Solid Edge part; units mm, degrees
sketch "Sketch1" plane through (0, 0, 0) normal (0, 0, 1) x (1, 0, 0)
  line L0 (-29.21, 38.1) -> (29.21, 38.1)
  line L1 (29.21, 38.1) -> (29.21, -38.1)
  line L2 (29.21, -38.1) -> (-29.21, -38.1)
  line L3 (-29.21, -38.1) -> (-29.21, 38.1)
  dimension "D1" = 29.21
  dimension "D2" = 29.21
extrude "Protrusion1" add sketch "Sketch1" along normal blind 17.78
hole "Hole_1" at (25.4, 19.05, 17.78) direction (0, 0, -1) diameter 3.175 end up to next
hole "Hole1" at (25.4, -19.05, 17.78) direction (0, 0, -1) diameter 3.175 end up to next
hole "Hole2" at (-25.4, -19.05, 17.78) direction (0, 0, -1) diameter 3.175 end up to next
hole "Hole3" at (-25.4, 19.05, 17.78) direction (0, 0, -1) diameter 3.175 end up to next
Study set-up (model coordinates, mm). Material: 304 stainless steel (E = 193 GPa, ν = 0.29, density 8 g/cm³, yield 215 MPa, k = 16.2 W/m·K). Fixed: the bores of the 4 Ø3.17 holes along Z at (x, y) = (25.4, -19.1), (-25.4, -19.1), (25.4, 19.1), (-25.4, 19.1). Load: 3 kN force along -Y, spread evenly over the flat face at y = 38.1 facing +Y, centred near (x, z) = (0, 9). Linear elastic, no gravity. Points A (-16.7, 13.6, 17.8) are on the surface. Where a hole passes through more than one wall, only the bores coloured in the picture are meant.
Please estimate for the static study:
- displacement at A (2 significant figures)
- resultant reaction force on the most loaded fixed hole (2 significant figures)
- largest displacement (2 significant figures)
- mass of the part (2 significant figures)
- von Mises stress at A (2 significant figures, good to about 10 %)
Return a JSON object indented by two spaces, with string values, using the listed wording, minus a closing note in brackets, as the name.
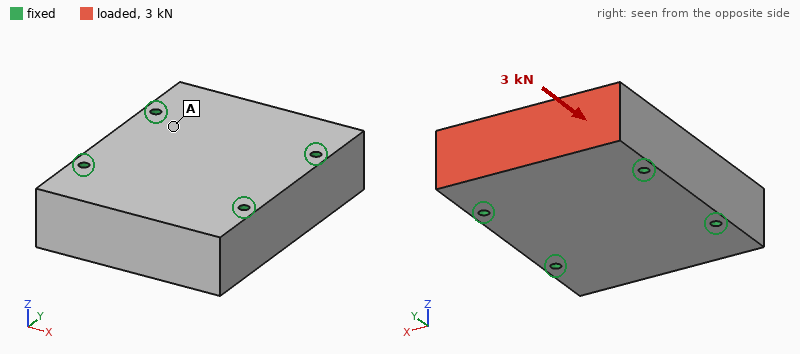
{
  "displacement at A": "0.23 µm",
  "resultant reaction force on the most loaded fixed hole": "1.1 kN",
  "largest displacement": "0.62 µm",
  "mass of the part": "630 g",
  "von Mises stress at A": "2.1 MPa"
}
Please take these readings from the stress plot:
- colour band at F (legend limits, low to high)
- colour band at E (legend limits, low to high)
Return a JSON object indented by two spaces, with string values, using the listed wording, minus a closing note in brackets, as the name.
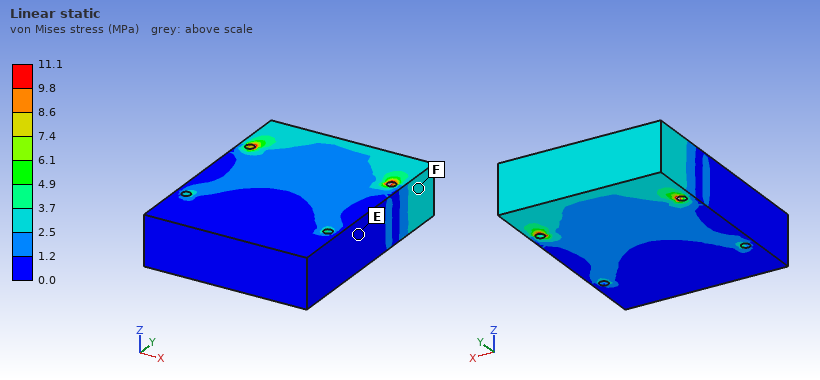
{
  "colour band at F": "2.5 to 3.7 MPa",
  "colour band at E": "0.0 to 1.2 MPa"
}
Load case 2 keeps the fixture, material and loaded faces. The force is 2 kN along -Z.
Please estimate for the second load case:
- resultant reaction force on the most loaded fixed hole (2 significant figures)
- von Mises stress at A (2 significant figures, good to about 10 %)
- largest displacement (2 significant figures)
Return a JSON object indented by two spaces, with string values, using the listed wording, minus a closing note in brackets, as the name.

{
  "resultant reaction force on the most loaded fixed hole": "1.2 kN",
  "von Mises stress at A": "6.7 MPa",
  "largest displacement": "3.6 µm"
}
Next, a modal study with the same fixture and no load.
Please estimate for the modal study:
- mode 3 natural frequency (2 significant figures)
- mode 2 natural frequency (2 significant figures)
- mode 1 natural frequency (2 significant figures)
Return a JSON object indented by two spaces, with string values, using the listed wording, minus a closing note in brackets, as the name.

{
  "mode 3 natural frequency": "20 kHz",
  "mode 2 natural frequency": "15 kHz",
  "mode 1 natural frequency": "14 kHz"
}
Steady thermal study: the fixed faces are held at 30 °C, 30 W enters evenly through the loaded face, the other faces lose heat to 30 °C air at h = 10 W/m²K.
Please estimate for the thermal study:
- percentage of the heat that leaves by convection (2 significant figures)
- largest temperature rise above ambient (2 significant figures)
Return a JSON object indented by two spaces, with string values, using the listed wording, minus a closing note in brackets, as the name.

{
  "percentage of the heat that leaves by convection": "4.4 %",
  "largest temperature rise above ambient": "50 K"
}
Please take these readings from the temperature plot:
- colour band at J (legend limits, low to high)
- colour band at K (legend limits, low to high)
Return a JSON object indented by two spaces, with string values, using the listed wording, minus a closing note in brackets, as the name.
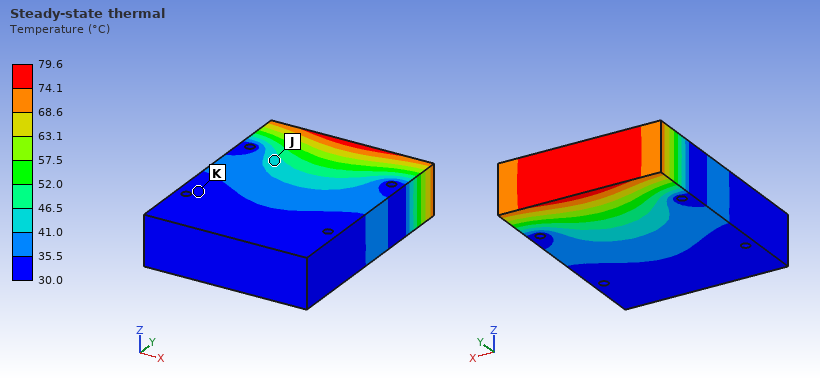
{
  "colour band at J": "41.0 to 46.5 °C",
  "colour band at K": "30.0 to 35.5 °C"
}
